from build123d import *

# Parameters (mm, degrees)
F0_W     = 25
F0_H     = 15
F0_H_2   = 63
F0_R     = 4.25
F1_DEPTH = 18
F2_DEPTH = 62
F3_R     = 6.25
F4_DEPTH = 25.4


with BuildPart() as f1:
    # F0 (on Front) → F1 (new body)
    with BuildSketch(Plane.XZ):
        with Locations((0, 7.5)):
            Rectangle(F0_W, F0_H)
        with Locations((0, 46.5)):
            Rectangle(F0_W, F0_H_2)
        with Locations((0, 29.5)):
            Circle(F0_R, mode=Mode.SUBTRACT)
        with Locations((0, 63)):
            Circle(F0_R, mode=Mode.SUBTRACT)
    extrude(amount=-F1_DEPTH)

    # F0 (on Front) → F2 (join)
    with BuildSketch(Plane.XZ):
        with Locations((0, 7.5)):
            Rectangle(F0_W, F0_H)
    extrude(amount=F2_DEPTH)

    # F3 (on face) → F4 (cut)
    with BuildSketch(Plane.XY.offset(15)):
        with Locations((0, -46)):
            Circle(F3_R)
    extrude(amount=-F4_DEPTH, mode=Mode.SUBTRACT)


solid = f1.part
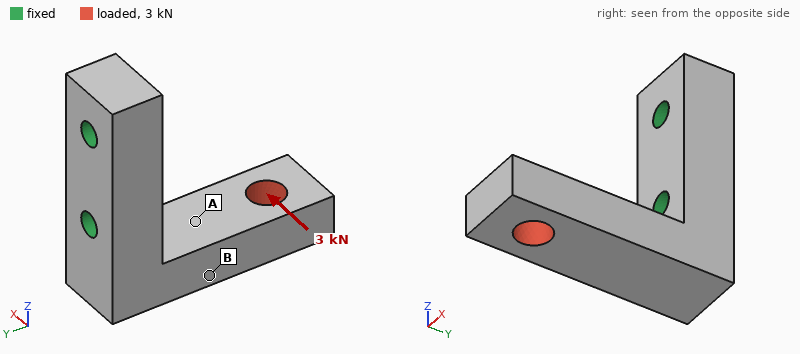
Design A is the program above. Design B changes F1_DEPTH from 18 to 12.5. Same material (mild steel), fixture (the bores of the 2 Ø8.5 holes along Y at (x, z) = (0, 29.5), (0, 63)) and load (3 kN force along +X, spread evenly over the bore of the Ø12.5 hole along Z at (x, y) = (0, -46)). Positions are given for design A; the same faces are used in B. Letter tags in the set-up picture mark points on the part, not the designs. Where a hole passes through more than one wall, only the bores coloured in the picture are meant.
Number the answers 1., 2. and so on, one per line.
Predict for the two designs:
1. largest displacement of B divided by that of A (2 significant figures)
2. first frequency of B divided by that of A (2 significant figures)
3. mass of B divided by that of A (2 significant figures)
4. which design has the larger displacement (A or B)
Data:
1. 1.5
2. 0.78
3. 0.81
4. B
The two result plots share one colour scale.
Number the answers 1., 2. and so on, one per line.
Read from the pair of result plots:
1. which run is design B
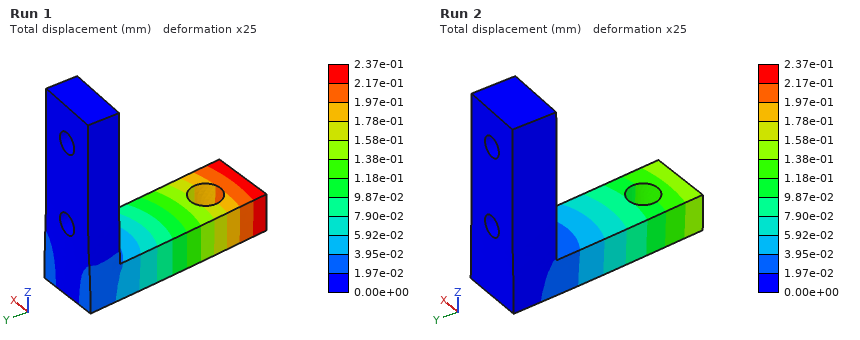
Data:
1. Run 1
